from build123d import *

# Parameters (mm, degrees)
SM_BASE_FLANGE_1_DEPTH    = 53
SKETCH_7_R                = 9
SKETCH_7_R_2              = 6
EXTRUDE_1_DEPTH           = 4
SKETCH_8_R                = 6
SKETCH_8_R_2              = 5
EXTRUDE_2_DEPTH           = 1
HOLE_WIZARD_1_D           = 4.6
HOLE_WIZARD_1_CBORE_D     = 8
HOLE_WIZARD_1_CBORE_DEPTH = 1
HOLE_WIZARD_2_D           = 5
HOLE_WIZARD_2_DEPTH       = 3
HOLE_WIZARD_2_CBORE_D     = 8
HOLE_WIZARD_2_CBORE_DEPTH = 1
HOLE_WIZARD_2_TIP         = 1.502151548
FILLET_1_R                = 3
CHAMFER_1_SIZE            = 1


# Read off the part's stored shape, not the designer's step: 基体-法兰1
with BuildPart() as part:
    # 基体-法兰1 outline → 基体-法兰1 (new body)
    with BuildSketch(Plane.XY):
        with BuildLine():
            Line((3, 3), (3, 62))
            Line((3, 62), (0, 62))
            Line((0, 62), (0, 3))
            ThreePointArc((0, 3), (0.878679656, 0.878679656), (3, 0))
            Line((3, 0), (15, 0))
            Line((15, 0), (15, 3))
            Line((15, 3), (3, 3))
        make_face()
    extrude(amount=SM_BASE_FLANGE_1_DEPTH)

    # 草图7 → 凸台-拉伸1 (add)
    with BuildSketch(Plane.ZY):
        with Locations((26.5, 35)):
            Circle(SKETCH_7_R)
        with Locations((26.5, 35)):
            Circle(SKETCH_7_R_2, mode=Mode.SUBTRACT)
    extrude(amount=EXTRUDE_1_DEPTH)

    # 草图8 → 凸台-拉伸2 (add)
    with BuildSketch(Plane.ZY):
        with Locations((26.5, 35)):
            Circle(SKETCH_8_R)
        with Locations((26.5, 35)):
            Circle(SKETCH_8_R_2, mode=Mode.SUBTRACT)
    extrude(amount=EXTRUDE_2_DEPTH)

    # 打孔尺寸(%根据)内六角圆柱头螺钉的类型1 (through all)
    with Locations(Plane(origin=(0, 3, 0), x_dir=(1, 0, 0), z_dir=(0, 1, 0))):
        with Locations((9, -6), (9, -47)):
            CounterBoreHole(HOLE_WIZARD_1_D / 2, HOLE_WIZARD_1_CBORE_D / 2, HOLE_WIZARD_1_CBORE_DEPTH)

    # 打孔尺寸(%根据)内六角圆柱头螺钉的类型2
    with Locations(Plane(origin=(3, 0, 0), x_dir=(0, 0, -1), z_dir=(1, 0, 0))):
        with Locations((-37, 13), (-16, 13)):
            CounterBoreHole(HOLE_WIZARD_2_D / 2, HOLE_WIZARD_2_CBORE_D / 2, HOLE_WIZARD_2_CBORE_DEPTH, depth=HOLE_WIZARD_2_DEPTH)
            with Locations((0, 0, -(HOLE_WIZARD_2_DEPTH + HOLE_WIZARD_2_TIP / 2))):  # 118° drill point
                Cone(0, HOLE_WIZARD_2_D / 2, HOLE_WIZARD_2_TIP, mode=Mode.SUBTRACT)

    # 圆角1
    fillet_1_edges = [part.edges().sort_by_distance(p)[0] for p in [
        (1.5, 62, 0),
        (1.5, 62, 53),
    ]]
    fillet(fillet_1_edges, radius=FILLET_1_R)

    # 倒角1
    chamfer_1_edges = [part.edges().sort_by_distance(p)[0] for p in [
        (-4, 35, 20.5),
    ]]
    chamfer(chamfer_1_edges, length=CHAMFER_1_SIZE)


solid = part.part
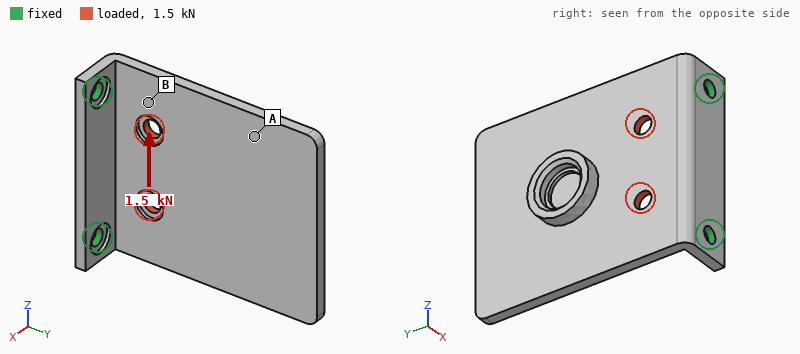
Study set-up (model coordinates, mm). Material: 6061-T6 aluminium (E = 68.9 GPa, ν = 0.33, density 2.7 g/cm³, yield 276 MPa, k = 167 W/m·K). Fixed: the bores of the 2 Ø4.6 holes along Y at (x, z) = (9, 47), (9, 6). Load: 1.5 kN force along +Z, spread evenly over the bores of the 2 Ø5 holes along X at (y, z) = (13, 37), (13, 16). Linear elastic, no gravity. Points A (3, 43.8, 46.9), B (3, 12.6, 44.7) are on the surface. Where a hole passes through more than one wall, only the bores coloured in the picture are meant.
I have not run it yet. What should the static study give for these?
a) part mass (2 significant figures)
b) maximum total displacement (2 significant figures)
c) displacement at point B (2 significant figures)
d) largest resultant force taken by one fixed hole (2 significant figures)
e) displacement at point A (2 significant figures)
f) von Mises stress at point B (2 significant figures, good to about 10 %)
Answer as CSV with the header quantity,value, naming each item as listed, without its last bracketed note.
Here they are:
quantity,value
part mass,32 g
maximum total displacement,87 µm
displacement at point B,33 µm
largest resultant force taken by one fixed hole,900 N
displacement at point A,67 µm
von Mises stress at point B,22 MPa
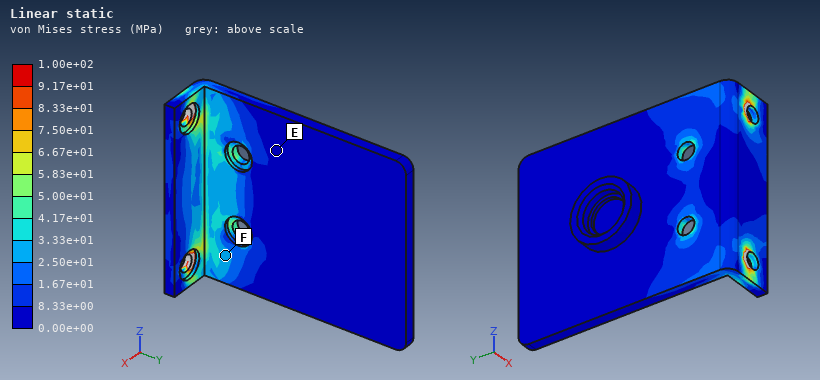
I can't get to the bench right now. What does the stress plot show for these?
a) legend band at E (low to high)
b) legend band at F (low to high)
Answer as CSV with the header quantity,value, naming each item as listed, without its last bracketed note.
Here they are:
quantity,value
legend band at E,0.00e+00 to 8.33e+00 MPa
legend band at F,2.50e+01 to 3.33e+01 MPa
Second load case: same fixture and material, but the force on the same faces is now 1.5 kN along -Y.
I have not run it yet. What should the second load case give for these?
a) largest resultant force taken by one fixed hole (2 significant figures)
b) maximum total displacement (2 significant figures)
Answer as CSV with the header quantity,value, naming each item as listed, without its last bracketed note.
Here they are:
quantity,value
largest resultant force taken by one fixed hole,760 N
maximum total displacement,0.72 mm
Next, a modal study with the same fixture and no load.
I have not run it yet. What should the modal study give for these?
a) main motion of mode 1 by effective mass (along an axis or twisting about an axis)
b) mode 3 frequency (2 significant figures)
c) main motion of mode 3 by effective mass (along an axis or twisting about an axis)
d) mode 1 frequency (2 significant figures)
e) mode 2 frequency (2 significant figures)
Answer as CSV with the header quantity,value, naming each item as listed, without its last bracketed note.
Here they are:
quantity,value
main motion of mode 1 by effective mass,along X
mode 3 frequency,3200 Hz
main motion of mode 3 by effective mass,along Z
mode 1 frequency,480 Hz
mode 2 frequency,1700 Hz
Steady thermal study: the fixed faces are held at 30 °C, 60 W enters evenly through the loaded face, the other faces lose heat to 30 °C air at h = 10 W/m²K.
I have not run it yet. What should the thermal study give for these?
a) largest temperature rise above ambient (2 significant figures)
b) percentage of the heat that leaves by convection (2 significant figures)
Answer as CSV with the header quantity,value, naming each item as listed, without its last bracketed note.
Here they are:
quantity,value
largest temperature rise above ambient,68 K
percentage of the heat that leaves by convection,6.6 %
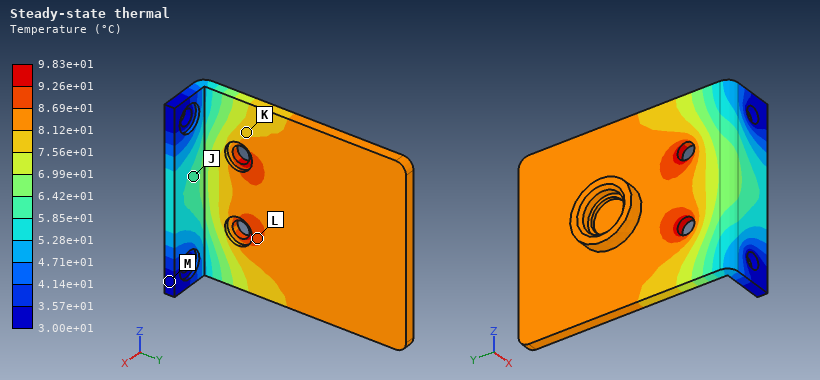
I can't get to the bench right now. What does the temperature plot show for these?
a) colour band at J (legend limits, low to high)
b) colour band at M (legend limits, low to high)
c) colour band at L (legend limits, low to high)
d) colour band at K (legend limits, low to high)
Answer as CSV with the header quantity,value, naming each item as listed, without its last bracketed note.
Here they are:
quantity,value
colour band at J,5.85e+01 to 6.42e+01 °C
colour band at M,3.00e+01 to 3.57e+01 °C
colour band at L,8.69e+01 to 9.26e+01 °C
colour band at K,7.56e+01 to 8.12e+01 °C
